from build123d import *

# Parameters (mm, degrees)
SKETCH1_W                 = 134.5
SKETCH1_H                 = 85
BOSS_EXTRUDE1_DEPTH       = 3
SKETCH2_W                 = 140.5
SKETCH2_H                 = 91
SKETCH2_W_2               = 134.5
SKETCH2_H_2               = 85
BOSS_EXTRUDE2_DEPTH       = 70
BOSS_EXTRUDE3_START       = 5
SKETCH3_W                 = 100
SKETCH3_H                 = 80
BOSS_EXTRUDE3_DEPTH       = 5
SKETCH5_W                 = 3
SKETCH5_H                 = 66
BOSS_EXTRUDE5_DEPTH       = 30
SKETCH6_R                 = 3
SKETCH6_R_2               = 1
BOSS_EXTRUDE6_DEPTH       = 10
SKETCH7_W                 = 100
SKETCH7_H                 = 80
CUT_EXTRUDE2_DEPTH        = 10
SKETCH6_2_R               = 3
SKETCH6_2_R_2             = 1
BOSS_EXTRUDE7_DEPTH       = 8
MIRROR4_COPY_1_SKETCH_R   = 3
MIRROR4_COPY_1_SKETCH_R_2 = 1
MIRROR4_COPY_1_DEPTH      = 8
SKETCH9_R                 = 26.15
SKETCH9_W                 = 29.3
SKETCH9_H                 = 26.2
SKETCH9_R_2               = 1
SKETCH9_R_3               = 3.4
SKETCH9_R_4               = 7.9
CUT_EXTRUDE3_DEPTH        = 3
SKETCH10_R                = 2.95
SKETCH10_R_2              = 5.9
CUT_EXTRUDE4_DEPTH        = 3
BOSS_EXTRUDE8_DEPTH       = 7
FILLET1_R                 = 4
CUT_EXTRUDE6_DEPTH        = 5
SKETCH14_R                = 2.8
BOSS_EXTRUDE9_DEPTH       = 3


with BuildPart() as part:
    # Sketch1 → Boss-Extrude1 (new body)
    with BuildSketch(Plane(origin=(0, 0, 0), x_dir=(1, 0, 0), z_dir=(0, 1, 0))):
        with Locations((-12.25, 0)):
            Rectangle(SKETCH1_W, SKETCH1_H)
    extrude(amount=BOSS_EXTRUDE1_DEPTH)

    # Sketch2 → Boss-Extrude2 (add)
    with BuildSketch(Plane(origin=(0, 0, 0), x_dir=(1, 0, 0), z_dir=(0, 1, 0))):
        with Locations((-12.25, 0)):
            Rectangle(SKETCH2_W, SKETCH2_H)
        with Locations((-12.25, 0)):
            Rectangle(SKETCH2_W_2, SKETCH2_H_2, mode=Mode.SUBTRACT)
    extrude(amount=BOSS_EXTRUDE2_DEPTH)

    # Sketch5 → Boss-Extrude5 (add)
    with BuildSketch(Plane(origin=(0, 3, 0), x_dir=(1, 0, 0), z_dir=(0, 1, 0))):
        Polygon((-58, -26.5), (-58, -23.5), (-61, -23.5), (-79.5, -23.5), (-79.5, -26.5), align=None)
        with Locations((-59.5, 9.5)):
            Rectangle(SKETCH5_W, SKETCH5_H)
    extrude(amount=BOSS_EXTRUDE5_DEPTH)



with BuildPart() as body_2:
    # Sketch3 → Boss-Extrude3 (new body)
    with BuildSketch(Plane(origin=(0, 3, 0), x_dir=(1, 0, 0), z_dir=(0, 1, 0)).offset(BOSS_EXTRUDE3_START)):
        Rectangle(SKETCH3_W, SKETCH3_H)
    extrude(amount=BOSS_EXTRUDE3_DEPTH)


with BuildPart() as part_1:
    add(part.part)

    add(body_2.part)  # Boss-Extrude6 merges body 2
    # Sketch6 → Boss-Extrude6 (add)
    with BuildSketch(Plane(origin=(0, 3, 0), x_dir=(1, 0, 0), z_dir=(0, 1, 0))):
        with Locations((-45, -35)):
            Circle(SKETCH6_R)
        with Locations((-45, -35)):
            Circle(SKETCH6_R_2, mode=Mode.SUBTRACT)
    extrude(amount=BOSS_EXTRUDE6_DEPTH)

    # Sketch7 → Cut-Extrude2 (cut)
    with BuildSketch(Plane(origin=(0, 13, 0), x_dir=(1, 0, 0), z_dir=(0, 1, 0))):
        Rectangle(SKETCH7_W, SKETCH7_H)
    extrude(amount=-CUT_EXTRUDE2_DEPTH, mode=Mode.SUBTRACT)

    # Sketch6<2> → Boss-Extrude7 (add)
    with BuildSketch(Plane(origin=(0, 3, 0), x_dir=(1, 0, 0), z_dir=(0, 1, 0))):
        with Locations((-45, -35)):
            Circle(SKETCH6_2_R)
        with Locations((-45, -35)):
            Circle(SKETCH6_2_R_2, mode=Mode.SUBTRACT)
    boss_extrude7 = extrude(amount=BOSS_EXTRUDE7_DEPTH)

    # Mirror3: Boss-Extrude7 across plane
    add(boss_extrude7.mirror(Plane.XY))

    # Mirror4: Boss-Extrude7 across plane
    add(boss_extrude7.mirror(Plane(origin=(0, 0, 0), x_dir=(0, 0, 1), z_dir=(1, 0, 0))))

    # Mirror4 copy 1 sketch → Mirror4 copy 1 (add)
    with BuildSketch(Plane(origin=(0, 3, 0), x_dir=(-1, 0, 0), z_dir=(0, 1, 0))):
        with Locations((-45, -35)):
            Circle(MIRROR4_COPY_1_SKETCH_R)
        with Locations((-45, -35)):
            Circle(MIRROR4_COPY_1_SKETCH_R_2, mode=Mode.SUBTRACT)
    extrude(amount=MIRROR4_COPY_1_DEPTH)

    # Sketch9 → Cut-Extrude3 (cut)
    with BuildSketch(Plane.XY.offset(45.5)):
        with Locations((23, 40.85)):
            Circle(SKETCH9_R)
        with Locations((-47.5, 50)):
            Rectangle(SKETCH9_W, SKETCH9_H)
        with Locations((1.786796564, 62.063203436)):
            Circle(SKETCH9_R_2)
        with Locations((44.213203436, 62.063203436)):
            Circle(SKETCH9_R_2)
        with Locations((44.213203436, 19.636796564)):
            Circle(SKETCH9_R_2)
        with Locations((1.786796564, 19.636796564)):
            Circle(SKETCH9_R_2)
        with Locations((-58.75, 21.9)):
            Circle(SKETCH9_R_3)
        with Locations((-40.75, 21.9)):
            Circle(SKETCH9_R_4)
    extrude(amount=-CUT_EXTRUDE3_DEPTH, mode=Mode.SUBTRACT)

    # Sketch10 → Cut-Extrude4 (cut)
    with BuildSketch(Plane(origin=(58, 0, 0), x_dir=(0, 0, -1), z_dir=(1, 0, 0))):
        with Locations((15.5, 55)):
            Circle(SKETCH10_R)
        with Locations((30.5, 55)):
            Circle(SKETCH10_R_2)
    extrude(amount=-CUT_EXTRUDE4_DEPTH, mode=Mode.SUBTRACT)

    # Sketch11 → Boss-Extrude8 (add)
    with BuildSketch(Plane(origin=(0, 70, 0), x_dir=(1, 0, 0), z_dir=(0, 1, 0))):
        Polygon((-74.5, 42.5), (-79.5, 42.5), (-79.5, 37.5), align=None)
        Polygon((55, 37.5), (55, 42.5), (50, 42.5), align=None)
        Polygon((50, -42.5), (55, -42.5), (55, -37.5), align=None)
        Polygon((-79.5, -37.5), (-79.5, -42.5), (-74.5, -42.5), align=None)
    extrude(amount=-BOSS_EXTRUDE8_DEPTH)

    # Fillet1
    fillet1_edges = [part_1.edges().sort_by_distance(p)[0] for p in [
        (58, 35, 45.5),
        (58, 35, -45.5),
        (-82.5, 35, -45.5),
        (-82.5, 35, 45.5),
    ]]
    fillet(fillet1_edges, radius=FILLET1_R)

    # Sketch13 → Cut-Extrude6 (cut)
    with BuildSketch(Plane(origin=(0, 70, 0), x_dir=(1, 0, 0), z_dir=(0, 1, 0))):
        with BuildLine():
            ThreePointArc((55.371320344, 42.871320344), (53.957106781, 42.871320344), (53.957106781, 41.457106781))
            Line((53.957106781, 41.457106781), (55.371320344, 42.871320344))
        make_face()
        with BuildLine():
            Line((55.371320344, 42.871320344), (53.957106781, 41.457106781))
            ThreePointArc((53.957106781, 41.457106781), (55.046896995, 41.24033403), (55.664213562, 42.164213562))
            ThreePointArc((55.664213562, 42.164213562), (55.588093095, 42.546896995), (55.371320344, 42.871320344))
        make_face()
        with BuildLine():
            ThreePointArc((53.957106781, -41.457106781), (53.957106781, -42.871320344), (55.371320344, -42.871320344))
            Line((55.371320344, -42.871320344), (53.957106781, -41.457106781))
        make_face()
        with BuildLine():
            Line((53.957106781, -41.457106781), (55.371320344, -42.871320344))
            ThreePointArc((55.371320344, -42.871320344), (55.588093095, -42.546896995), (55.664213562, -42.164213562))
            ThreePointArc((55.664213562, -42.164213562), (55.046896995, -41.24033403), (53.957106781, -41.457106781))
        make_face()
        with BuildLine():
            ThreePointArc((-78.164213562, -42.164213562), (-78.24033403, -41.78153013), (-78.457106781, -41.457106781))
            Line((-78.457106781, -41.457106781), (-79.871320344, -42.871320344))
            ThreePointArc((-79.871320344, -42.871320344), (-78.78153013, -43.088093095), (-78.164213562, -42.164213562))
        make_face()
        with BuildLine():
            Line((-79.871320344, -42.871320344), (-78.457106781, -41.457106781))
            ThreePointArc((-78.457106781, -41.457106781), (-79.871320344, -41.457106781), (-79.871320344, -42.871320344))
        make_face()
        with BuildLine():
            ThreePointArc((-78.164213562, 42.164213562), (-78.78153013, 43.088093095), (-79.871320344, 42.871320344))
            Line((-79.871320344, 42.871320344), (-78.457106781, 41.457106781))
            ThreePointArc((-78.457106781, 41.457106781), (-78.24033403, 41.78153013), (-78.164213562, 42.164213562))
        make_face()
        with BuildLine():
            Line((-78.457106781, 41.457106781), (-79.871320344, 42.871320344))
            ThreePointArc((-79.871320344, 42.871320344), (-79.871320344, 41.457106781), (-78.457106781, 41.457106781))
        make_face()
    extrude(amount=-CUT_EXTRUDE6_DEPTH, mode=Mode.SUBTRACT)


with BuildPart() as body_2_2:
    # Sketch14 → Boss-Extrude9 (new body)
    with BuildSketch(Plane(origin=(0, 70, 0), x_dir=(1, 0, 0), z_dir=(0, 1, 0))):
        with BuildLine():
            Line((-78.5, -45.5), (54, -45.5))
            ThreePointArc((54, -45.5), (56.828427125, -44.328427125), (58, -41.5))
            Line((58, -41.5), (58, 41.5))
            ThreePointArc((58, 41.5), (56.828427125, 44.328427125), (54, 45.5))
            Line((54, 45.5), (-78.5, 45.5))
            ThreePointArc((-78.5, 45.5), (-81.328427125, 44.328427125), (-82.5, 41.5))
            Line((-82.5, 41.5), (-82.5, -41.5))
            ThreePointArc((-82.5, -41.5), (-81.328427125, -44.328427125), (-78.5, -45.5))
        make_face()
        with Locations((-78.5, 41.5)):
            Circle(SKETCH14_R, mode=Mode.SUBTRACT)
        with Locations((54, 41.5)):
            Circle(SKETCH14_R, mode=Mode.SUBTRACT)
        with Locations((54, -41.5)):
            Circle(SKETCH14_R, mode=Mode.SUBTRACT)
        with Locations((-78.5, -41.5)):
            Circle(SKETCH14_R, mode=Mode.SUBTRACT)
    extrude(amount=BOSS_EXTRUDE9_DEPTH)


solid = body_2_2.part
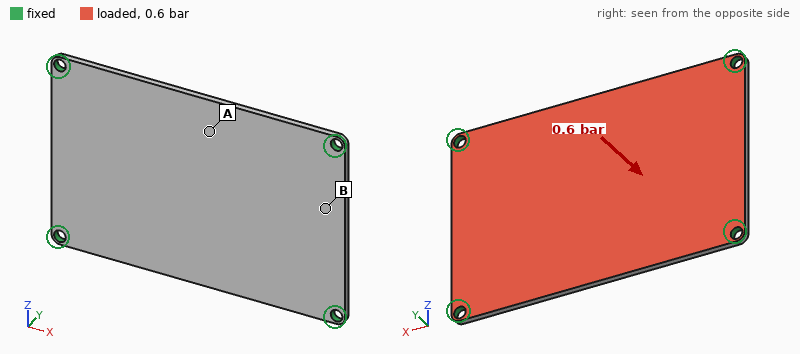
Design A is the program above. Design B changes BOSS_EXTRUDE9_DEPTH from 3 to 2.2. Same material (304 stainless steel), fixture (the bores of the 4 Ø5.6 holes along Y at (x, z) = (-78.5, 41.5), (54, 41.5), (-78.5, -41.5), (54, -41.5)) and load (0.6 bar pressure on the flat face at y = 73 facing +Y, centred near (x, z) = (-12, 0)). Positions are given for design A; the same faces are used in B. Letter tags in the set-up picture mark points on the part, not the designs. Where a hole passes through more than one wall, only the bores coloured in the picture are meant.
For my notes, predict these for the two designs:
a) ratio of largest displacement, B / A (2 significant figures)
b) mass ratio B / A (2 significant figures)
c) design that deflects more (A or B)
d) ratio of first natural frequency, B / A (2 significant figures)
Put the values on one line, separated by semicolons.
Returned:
2.5; 0.73; B; 0.74
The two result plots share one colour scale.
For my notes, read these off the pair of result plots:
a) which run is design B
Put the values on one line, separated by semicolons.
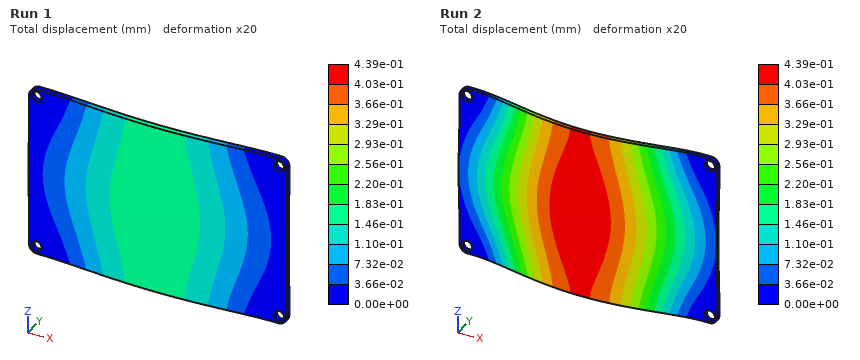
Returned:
Run 2
